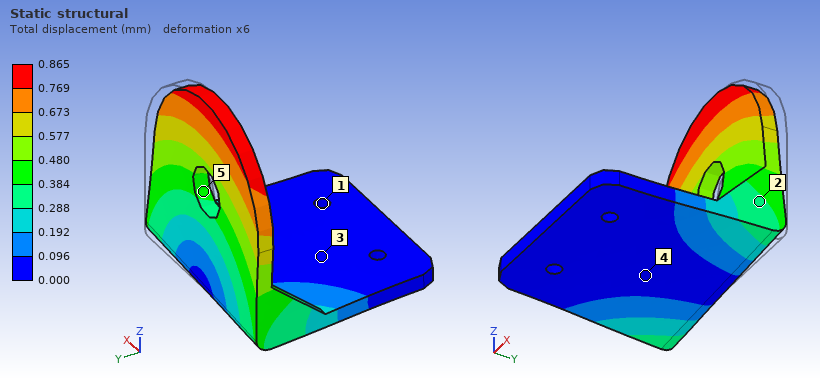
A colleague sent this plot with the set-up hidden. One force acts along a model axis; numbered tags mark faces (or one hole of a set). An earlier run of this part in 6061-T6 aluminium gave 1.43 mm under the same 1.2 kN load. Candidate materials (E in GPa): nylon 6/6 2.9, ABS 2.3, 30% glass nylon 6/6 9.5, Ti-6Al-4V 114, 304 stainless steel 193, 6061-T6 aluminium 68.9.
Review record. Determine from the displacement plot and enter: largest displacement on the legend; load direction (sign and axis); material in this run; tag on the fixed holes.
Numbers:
0.865 mm
-X
Ti-6Al-4V
1
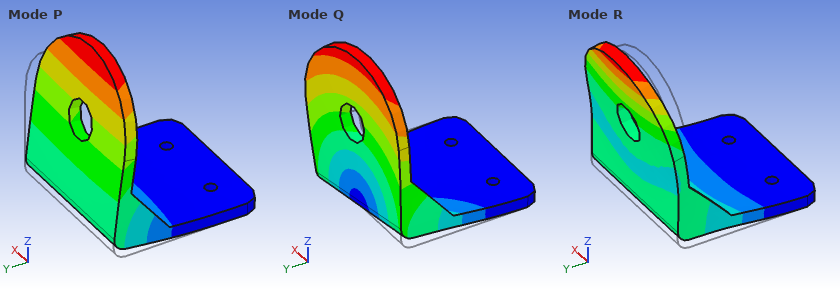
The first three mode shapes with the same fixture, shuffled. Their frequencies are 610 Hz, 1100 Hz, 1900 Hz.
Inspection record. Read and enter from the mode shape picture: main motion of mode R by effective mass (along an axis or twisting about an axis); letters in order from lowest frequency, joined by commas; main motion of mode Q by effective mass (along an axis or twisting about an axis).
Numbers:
along Z
P, Q, R
along X
